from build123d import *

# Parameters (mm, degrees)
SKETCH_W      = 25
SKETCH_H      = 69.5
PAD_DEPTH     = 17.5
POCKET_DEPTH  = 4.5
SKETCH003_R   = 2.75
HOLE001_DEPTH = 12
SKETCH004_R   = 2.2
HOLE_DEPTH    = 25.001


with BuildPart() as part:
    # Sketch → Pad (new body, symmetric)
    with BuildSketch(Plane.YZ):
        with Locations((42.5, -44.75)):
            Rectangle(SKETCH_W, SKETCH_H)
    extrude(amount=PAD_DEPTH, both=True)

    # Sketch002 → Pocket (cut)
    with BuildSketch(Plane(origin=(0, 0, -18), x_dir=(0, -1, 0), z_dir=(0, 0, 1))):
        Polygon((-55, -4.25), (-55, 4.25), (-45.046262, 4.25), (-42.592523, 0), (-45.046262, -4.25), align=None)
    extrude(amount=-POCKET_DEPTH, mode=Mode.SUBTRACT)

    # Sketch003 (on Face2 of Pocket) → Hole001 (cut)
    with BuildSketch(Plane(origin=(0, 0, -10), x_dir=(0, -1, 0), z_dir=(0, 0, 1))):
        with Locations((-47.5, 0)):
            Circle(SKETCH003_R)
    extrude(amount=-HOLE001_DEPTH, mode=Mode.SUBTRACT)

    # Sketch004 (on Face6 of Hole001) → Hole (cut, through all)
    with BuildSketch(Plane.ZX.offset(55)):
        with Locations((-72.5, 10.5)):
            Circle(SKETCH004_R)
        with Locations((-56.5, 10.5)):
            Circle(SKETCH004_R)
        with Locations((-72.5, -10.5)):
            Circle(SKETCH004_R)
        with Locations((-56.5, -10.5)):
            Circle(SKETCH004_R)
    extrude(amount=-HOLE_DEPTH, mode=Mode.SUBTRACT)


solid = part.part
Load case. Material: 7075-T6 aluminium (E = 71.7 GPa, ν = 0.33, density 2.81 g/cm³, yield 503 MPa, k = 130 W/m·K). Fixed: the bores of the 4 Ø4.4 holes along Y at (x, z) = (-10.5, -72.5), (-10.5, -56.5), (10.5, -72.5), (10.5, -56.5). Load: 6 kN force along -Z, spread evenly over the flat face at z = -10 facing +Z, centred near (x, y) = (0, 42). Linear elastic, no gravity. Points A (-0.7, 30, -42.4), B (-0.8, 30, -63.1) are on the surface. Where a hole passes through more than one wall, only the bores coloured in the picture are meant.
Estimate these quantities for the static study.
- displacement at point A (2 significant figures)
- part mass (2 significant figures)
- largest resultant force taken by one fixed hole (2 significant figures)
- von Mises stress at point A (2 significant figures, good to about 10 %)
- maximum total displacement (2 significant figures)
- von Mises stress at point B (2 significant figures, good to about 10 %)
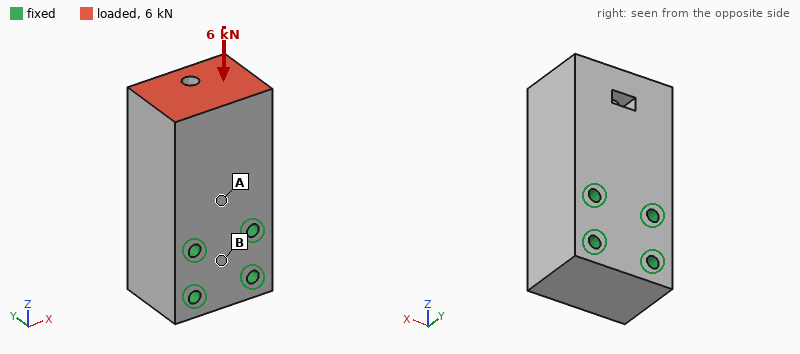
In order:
1.6 µm
160 g
2.6 kN
6.3 MPa
5.7 µm
2.4 MPa
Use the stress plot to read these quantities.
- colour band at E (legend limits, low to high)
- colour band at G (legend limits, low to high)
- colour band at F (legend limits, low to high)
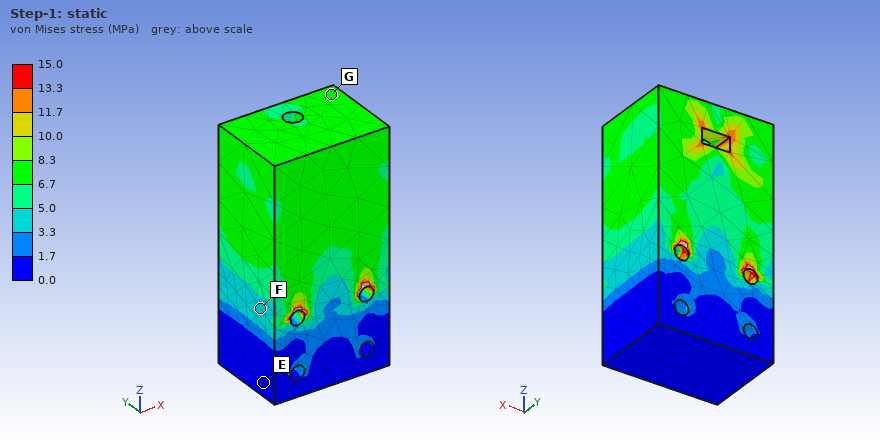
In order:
0.0 to 1.7 MPa
6.7 to 8.3 MPa
3.3 to 5.0 MPa
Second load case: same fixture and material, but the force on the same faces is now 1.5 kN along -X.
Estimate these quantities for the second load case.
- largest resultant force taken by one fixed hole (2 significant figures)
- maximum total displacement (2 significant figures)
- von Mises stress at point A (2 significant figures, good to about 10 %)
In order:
2.7 kN
14 µm
4.9 MPa
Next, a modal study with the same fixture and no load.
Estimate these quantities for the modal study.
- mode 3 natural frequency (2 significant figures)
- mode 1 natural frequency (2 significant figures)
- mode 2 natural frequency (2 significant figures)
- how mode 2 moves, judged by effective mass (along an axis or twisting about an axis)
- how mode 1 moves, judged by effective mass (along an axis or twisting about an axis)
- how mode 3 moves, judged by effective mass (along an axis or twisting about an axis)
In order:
15 kHz
7700 Hz
9600 Hz
along X
along Y
twisting about Z
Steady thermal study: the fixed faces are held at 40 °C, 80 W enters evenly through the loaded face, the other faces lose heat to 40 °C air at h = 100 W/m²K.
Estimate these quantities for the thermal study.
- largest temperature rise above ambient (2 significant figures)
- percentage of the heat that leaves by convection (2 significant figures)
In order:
32 K
12 %
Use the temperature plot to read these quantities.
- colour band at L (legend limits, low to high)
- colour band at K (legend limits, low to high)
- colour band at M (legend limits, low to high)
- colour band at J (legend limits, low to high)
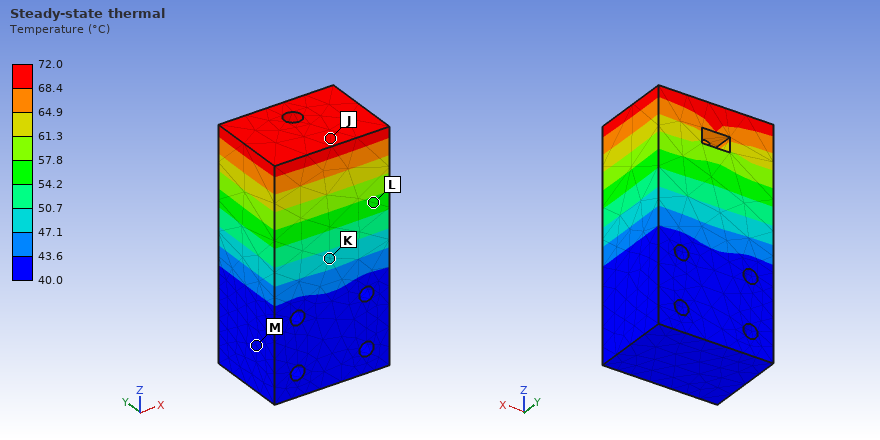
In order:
54.2 to 57.8 °C
47.1 to 50.7 °C
40.0 to 43.6 °C
68.4 to 72.0 °C
